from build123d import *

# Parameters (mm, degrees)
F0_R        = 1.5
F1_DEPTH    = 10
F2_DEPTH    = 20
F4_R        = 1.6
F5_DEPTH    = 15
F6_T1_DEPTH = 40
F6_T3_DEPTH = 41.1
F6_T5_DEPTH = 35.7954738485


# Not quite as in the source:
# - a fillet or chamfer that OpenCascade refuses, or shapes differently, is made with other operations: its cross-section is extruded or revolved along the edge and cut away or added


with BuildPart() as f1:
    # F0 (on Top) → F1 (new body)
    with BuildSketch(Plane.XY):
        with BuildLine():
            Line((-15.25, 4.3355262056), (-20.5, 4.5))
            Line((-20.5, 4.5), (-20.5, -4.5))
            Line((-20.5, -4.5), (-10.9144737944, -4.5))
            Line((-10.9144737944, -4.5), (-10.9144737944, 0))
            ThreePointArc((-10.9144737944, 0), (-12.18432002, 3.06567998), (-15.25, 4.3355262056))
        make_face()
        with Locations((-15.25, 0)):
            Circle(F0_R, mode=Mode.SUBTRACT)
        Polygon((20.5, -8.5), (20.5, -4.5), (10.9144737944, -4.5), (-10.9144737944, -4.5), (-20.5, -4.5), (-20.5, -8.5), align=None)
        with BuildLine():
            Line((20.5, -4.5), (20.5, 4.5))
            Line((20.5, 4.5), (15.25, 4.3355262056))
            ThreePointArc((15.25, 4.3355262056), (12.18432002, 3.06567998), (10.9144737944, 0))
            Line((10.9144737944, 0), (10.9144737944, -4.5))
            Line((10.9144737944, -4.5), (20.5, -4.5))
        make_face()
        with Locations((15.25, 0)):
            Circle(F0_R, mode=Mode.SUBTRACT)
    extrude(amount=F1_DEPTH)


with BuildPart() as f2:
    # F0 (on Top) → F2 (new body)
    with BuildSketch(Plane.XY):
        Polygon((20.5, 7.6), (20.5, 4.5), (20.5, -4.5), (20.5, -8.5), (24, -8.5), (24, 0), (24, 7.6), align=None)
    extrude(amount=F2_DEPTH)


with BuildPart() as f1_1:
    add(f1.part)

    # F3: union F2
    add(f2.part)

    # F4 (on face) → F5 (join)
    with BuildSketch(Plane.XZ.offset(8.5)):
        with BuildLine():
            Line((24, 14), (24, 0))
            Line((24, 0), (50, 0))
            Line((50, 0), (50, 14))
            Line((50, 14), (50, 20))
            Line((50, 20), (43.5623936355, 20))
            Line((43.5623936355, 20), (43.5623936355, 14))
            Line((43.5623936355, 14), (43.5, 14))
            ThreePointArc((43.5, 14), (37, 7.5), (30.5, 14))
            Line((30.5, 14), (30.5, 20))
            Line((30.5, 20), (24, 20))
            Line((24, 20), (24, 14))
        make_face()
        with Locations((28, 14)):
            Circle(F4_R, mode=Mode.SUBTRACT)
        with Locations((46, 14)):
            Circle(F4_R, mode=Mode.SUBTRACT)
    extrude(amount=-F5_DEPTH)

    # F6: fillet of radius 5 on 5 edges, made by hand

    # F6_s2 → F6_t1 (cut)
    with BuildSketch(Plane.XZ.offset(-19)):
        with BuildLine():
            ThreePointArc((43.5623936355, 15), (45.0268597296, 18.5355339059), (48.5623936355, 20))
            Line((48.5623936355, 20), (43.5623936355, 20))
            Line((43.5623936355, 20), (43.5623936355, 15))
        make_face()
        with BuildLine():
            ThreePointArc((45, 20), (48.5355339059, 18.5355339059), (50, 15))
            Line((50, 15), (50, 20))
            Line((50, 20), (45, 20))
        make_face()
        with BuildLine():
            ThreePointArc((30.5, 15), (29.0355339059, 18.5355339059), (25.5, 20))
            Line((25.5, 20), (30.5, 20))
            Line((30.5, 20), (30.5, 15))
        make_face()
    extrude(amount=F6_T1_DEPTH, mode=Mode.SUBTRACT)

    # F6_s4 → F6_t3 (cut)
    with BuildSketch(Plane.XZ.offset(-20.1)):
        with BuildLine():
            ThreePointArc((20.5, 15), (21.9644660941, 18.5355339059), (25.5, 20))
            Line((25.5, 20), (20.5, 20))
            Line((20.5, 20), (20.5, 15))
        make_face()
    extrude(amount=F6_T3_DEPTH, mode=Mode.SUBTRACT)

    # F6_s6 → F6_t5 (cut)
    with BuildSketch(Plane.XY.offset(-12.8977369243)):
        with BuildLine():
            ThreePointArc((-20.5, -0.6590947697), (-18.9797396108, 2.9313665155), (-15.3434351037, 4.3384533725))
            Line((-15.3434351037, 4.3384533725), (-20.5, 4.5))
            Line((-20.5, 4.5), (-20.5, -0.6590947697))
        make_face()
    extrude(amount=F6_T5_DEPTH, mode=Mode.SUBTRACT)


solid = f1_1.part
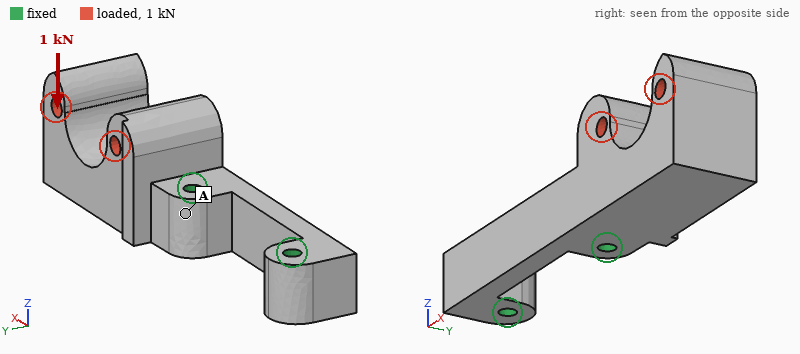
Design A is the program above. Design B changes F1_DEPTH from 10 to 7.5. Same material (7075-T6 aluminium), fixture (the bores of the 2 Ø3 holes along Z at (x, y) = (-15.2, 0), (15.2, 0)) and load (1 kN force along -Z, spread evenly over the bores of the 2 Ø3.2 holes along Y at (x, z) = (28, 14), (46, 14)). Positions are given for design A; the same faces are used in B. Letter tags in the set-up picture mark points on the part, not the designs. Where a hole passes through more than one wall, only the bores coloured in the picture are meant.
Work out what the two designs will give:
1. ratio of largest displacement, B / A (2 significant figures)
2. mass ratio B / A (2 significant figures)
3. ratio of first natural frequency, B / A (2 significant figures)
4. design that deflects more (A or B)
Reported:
1.9
0.92
0.77
B
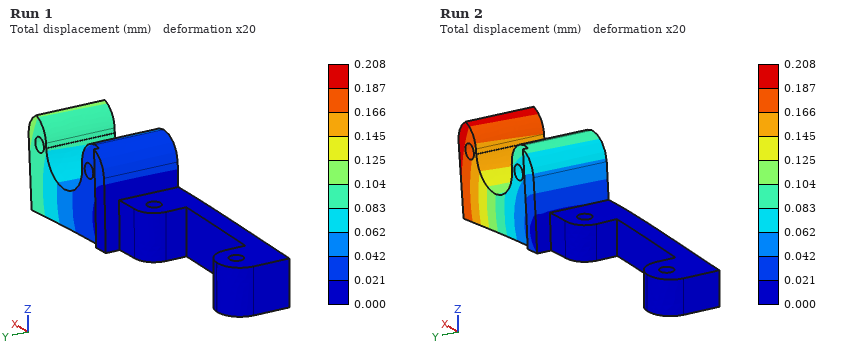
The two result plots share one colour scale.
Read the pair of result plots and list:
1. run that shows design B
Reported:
Run 2
